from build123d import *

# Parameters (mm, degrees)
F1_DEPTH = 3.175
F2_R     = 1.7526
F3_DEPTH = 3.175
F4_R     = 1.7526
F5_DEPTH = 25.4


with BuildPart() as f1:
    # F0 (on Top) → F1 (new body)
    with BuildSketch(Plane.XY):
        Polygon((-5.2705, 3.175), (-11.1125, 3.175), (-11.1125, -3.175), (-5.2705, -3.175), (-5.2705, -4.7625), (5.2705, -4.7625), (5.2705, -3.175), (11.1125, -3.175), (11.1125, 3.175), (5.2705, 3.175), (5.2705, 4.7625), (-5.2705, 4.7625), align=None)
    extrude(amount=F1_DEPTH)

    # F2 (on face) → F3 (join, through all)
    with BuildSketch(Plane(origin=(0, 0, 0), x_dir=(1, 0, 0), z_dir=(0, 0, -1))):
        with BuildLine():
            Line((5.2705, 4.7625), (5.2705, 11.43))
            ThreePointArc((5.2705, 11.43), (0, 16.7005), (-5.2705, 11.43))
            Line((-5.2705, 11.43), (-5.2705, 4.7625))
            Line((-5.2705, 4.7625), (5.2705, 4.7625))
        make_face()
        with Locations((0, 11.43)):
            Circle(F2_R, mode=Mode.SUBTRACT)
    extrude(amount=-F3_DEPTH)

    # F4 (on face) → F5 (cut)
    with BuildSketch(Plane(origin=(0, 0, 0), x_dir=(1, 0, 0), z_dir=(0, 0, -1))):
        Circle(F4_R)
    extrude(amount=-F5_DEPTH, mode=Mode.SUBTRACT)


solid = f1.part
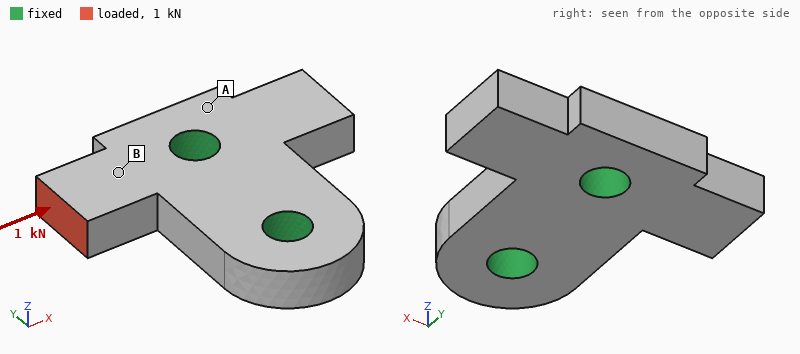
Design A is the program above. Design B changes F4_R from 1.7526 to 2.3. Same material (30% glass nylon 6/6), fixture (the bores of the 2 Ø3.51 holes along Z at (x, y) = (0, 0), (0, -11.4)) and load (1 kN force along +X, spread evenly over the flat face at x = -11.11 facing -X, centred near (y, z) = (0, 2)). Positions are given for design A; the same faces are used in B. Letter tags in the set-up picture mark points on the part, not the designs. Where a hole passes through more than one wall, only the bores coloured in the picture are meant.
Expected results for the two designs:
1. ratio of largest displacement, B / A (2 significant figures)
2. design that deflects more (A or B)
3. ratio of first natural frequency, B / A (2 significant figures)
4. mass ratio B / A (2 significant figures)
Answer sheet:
0.90
A
1.1
0.97
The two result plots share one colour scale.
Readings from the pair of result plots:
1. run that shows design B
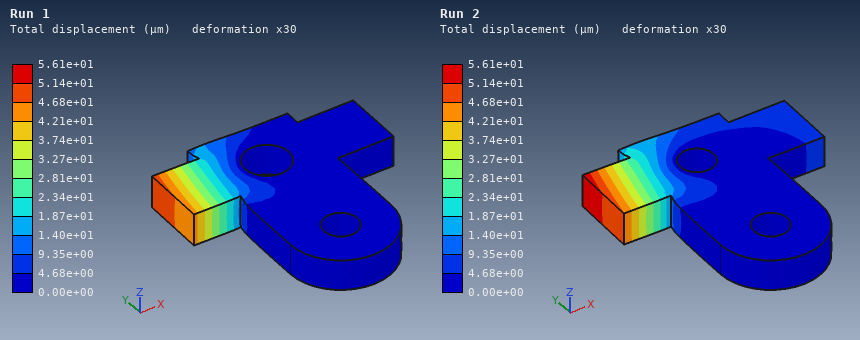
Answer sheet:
Run 1
